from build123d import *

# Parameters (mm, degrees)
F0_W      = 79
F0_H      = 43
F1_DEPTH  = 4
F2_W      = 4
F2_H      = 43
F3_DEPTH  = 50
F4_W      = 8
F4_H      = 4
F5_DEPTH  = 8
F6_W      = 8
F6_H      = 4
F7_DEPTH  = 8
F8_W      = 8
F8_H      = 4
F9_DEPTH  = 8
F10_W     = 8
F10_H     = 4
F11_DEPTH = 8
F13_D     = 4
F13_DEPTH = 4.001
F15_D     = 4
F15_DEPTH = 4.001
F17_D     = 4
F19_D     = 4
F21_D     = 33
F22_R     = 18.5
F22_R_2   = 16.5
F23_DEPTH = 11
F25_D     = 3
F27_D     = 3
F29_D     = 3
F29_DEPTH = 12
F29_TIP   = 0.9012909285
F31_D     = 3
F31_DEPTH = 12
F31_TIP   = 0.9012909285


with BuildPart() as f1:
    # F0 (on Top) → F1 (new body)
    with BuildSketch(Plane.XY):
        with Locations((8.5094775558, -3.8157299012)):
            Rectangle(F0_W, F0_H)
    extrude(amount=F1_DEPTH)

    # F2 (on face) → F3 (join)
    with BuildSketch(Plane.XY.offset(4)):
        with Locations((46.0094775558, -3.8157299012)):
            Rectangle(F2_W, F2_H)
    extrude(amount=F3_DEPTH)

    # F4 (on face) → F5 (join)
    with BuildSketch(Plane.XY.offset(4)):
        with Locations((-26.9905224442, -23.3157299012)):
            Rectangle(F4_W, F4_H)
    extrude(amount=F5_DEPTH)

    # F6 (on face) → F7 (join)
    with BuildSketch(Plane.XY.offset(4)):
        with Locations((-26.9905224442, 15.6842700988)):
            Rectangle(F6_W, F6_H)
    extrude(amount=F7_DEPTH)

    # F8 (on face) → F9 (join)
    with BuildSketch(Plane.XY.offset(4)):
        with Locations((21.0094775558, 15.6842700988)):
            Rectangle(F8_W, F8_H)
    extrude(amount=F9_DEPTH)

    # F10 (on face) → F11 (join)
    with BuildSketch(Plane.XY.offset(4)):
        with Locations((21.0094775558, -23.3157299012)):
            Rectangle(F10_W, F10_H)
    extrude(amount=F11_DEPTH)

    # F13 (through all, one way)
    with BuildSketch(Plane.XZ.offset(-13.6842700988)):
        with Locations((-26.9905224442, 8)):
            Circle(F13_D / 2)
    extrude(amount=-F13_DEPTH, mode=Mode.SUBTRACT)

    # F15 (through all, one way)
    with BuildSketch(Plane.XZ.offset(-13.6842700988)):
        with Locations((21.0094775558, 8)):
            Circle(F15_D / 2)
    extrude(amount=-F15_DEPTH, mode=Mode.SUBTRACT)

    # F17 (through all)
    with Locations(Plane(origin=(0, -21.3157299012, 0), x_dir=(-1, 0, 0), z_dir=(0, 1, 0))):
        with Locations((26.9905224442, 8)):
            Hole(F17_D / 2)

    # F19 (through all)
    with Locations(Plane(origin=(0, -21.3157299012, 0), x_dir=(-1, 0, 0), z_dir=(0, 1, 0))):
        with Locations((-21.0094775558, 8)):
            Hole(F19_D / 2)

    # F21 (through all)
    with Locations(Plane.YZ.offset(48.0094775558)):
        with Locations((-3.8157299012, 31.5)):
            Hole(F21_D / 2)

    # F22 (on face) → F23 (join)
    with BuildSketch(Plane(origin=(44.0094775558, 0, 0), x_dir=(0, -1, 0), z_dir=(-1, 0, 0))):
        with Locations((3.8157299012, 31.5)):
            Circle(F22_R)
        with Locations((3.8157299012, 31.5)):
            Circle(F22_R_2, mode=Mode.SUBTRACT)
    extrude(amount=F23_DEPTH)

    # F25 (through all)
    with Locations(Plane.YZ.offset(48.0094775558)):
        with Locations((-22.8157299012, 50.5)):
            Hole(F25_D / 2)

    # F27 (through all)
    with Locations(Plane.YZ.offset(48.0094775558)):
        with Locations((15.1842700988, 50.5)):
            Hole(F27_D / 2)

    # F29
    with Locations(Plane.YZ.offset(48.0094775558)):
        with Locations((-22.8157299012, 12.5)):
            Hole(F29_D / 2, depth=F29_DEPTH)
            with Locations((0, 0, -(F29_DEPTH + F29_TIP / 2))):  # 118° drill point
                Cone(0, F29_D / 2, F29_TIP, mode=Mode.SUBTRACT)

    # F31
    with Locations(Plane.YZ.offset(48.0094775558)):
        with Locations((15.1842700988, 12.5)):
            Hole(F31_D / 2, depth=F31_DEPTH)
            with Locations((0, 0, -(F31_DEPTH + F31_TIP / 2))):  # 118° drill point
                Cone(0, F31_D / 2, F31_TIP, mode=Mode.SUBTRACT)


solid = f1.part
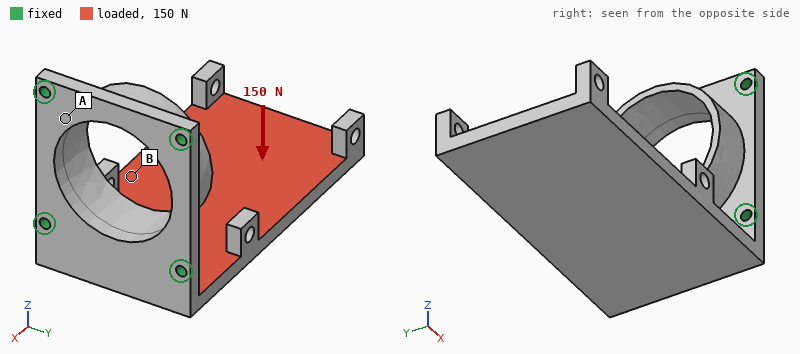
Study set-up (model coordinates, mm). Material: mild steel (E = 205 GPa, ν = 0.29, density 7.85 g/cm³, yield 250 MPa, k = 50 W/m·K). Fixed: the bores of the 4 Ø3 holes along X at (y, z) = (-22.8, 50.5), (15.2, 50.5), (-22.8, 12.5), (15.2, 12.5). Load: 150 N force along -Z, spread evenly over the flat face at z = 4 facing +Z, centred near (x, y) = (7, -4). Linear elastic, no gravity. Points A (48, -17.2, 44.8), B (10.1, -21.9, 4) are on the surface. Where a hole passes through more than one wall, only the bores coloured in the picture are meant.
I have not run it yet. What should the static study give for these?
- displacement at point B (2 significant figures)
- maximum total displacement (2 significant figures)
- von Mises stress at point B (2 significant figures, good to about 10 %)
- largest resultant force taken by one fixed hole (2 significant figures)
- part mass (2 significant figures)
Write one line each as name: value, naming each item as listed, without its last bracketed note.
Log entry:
displacement at point B: 0.10 mm
maximum total displacement: 0.28 mm
von Mises stress at point B: 15 MPa
largest resultant force taken by one fixed hole: 130 N
part mass: 170 g
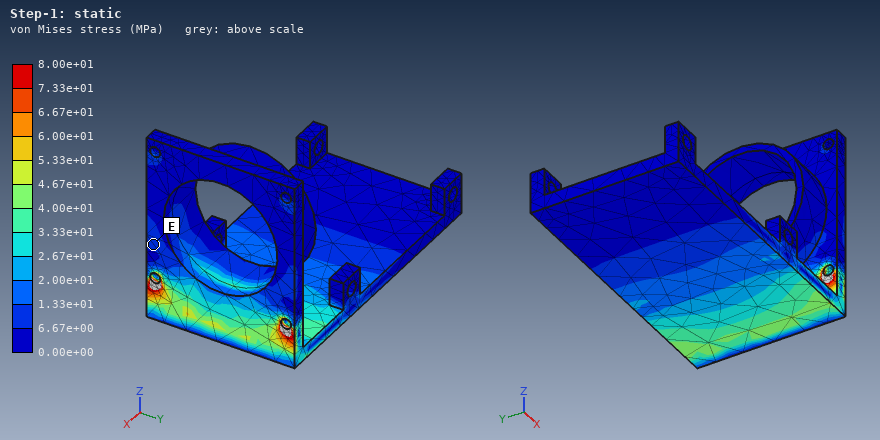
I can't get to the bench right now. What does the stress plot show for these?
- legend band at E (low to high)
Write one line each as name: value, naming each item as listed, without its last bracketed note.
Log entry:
legend band at E: 6.67e+00 to 1.33e+01 MPa
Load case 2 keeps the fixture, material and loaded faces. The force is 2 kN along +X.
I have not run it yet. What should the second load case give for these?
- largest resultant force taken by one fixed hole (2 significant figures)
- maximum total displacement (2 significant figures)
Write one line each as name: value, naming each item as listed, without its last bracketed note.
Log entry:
largest resultant force taken by one fixed hole: 1.1 kN
maximum total displacement: 47 µm
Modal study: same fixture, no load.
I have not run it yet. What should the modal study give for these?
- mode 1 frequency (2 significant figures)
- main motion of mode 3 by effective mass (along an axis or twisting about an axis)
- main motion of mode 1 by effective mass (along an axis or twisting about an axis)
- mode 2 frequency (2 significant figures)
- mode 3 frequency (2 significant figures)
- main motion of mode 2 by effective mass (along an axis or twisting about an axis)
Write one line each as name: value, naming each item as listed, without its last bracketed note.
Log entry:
mode 1 frequency: 430 Hz
main motion of mode 3 by effective mass: along Y
main motion of mode 1 by effective mass: along Z
mode 2 frequency: 1600 Hz
mode 3 frequency: 2100 Hz
main motion of mode 2 by effective mass: along Y
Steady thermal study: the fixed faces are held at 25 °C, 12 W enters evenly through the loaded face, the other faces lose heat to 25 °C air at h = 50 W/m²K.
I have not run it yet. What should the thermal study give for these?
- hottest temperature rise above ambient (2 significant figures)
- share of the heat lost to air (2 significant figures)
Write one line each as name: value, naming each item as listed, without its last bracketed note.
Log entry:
hottest temperature rise above ambient: 31 K
share of the heat lost to air: 58 %
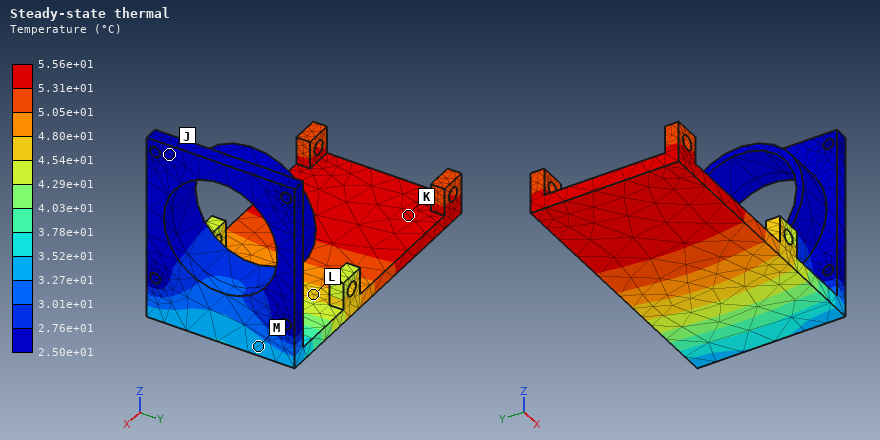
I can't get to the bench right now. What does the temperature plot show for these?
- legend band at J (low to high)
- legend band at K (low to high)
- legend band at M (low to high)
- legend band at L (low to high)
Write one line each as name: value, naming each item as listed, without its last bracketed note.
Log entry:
legend band at J: 2.50e+01 to 2.76e+01 °C
legend band at K: 5.31e+01 to 5.56e+01 °C
legend band at M: 3.27e+01 to 3.52e+01 °C
legend band at L: 4.54e+01 to 4.80e+01 °C
